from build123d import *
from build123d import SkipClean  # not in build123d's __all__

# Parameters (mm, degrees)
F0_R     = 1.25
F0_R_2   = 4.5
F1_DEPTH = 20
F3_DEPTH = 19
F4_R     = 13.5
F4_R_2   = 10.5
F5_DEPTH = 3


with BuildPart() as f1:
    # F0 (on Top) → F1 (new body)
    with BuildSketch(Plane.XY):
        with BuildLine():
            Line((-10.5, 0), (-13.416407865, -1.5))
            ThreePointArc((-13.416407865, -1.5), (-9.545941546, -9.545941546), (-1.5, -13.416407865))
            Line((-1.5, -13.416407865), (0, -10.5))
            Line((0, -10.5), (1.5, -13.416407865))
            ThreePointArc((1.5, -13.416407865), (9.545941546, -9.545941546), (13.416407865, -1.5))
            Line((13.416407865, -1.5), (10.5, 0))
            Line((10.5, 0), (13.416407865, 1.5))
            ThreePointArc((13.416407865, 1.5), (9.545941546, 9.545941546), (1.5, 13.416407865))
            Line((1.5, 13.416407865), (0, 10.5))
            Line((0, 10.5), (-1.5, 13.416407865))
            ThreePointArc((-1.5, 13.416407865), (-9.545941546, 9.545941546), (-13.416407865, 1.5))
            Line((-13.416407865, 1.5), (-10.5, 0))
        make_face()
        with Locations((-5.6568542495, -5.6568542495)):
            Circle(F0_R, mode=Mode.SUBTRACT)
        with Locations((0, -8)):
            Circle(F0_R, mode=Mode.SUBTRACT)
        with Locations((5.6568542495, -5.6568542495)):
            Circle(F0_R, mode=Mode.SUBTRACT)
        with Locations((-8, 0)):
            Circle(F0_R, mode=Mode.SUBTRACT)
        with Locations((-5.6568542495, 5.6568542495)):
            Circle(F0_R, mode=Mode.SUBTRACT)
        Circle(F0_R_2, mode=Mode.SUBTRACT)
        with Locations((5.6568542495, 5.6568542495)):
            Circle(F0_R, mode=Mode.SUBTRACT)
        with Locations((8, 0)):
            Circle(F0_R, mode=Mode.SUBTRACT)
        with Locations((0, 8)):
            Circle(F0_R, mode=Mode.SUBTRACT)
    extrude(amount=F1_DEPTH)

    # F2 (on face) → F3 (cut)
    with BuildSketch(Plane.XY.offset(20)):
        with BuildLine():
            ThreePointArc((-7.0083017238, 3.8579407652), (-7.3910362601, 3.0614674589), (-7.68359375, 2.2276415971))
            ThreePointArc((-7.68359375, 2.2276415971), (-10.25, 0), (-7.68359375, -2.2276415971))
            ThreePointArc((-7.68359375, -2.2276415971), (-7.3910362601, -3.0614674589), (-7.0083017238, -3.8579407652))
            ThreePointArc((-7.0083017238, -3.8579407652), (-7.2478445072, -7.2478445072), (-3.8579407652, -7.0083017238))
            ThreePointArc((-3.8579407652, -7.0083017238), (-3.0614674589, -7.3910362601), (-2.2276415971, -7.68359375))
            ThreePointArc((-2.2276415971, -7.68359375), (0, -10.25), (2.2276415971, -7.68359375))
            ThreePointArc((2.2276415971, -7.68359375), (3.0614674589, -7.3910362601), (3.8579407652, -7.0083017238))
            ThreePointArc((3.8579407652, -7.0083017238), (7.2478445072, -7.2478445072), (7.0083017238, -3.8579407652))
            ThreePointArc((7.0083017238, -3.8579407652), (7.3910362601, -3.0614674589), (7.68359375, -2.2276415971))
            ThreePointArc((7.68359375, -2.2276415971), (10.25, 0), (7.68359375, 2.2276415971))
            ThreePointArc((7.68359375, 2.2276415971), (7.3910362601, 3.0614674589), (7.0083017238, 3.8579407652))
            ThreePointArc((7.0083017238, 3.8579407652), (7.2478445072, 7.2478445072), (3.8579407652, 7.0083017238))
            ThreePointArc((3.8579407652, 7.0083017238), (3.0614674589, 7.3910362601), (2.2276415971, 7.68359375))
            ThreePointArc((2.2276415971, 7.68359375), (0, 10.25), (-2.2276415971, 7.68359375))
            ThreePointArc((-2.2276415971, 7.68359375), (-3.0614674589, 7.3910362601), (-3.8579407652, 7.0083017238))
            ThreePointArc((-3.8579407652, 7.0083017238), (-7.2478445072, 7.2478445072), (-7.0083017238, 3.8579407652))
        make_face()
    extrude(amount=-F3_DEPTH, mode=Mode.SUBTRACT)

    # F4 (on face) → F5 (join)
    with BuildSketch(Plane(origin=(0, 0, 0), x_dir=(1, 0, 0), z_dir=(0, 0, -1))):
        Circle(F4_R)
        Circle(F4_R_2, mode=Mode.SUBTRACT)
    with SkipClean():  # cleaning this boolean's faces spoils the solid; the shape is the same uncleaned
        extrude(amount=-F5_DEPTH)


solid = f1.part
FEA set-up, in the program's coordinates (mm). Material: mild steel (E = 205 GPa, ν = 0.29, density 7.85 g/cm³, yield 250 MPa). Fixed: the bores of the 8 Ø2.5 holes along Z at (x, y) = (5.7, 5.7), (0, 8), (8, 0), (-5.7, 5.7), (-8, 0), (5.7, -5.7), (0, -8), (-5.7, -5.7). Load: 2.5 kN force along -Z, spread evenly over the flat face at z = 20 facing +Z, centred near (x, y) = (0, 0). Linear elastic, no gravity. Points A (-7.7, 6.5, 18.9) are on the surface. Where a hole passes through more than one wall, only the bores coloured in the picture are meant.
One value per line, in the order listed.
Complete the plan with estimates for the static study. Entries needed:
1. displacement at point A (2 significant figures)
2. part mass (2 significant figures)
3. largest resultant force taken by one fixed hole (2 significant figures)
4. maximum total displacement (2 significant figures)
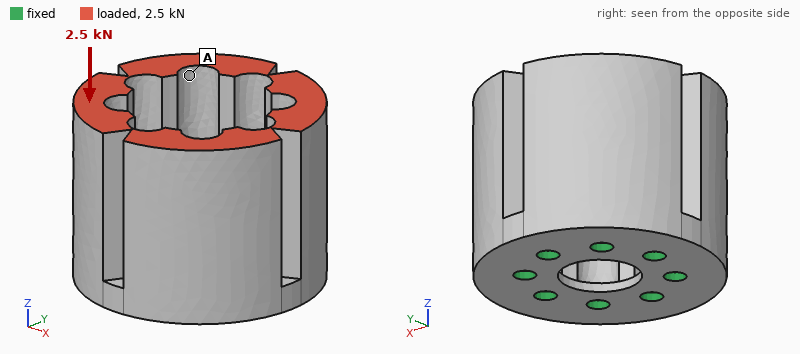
2.5 µm
47 g
330 N
2.7 µm
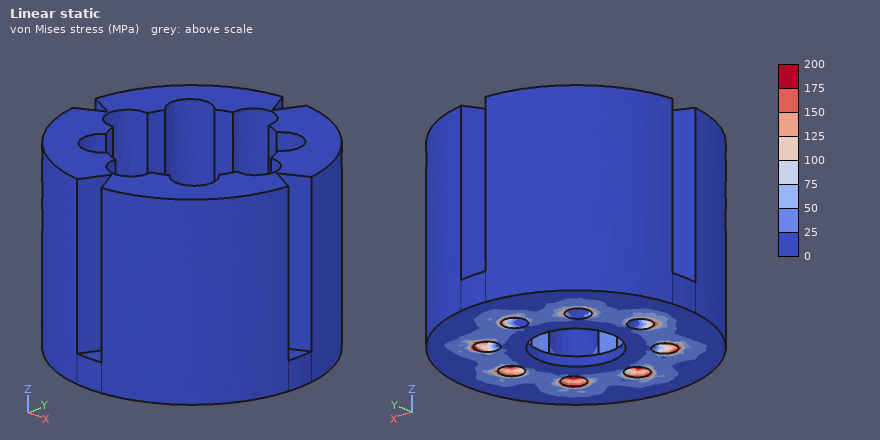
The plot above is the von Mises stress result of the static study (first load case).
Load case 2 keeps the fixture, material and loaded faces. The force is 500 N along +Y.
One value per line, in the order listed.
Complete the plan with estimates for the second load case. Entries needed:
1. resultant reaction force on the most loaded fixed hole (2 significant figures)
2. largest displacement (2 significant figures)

270 N
7.5 µm
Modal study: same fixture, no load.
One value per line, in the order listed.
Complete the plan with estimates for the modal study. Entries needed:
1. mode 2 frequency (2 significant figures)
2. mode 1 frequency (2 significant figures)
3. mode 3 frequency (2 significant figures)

10 kHz
10 kHz
14 kHz
